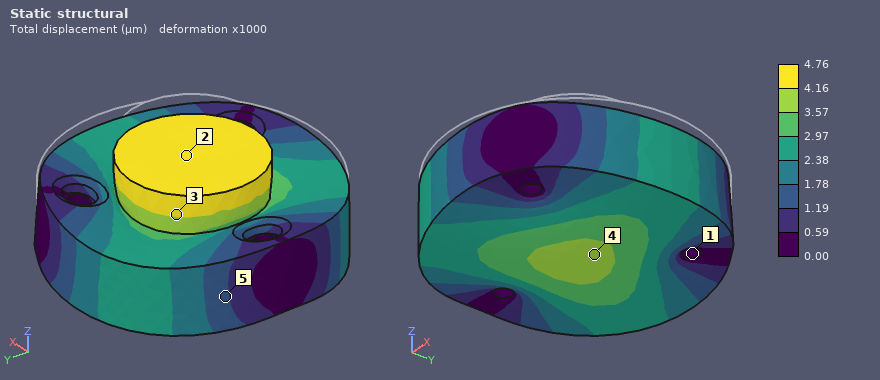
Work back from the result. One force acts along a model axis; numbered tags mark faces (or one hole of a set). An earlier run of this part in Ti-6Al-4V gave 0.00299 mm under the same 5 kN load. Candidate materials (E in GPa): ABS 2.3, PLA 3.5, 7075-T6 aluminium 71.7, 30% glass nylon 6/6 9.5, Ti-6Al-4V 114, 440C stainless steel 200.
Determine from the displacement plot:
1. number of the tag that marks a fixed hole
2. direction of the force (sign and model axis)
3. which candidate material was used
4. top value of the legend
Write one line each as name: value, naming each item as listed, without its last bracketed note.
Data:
number of the tag that marks a fixed hole: 1
direction of the force: -Z
which candidate material was used: 7075-T6 aluminium
top value of the legend: 4.76 µm
